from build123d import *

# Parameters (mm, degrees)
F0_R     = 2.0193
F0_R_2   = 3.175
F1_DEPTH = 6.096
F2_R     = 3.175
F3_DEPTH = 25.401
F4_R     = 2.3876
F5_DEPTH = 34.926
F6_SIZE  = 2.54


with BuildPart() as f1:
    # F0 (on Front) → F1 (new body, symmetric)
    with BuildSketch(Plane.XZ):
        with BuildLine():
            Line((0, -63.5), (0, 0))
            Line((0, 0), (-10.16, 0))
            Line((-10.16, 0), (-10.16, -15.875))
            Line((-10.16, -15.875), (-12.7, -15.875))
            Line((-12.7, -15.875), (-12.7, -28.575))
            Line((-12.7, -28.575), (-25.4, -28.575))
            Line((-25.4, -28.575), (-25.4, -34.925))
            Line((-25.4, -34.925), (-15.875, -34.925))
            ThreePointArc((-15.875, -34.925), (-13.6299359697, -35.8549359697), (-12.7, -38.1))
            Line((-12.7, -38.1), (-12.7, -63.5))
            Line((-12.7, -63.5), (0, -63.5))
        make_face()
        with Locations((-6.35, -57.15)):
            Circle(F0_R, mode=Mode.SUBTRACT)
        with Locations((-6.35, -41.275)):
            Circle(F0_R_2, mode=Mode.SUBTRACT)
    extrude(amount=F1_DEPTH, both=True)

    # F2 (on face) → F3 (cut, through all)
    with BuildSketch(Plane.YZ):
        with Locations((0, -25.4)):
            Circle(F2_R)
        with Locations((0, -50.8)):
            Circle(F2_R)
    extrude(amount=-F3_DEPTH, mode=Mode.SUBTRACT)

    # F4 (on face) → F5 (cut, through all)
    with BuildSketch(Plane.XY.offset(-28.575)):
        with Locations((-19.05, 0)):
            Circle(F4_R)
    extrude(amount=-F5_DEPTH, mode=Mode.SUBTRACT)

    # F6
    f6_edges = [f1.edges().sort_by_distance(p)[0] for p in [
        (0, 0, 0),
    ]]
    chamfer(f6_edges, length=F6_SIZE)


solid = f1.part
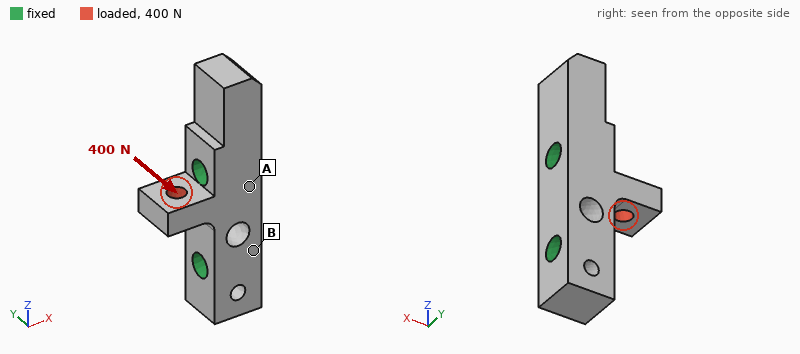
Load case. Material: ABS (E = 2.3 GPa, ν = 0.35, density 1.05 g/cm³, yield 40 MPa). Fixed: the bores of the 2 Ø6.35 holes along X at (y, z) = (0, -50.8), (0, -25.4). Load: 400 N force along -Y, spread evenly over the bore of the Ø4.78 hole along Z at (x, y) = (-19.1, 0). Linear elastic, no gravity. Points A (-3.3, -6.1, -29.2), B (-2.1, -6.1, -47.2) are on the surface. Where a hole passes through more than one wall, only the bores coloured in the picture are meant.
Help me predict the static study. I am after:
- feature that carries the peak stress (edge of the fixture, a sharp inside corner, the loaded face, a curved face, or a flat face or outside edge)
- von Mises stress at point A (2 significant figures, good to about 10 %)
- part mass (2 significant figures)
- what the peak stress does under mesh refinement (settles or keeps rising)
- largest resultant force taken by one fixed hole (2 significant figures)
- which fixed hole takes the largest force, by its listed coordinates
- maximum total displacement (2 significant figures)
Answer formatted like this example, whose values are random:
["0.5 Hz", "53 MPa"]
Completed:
["edge of the fixture", "5.6 MPa", "9.3 g", "keeps rising", "360 N", "(0, -25.4)", "0.29 mm"]
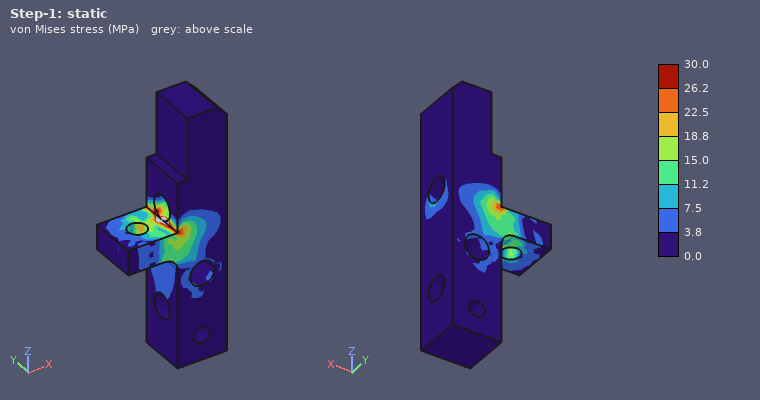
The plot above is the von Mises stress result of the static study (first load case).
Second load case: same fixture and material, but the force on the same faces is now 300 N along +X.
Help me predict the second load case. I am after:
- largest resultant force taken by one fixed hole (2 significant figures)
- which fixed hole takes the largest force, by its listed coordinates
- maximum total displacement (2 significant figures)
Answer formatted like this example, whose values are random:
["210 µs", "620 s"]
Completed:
["260 N", "(0, -25.4)", "39 µm"]
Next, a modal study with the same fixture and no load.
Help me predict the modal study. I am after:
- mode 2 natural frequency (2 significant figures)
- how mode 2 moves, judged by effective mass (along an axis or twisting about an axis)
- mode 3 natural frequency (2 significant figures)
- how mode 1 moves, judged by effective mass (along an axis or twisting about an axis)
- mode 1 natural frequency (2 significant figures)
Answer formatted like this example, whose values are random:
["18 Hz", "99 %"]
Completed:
["4700 Hz", "along X", "6600 Hz", "along Y", "4200 Hz"]
